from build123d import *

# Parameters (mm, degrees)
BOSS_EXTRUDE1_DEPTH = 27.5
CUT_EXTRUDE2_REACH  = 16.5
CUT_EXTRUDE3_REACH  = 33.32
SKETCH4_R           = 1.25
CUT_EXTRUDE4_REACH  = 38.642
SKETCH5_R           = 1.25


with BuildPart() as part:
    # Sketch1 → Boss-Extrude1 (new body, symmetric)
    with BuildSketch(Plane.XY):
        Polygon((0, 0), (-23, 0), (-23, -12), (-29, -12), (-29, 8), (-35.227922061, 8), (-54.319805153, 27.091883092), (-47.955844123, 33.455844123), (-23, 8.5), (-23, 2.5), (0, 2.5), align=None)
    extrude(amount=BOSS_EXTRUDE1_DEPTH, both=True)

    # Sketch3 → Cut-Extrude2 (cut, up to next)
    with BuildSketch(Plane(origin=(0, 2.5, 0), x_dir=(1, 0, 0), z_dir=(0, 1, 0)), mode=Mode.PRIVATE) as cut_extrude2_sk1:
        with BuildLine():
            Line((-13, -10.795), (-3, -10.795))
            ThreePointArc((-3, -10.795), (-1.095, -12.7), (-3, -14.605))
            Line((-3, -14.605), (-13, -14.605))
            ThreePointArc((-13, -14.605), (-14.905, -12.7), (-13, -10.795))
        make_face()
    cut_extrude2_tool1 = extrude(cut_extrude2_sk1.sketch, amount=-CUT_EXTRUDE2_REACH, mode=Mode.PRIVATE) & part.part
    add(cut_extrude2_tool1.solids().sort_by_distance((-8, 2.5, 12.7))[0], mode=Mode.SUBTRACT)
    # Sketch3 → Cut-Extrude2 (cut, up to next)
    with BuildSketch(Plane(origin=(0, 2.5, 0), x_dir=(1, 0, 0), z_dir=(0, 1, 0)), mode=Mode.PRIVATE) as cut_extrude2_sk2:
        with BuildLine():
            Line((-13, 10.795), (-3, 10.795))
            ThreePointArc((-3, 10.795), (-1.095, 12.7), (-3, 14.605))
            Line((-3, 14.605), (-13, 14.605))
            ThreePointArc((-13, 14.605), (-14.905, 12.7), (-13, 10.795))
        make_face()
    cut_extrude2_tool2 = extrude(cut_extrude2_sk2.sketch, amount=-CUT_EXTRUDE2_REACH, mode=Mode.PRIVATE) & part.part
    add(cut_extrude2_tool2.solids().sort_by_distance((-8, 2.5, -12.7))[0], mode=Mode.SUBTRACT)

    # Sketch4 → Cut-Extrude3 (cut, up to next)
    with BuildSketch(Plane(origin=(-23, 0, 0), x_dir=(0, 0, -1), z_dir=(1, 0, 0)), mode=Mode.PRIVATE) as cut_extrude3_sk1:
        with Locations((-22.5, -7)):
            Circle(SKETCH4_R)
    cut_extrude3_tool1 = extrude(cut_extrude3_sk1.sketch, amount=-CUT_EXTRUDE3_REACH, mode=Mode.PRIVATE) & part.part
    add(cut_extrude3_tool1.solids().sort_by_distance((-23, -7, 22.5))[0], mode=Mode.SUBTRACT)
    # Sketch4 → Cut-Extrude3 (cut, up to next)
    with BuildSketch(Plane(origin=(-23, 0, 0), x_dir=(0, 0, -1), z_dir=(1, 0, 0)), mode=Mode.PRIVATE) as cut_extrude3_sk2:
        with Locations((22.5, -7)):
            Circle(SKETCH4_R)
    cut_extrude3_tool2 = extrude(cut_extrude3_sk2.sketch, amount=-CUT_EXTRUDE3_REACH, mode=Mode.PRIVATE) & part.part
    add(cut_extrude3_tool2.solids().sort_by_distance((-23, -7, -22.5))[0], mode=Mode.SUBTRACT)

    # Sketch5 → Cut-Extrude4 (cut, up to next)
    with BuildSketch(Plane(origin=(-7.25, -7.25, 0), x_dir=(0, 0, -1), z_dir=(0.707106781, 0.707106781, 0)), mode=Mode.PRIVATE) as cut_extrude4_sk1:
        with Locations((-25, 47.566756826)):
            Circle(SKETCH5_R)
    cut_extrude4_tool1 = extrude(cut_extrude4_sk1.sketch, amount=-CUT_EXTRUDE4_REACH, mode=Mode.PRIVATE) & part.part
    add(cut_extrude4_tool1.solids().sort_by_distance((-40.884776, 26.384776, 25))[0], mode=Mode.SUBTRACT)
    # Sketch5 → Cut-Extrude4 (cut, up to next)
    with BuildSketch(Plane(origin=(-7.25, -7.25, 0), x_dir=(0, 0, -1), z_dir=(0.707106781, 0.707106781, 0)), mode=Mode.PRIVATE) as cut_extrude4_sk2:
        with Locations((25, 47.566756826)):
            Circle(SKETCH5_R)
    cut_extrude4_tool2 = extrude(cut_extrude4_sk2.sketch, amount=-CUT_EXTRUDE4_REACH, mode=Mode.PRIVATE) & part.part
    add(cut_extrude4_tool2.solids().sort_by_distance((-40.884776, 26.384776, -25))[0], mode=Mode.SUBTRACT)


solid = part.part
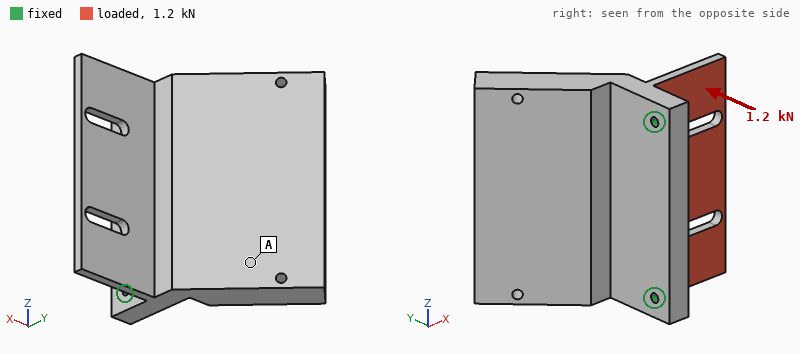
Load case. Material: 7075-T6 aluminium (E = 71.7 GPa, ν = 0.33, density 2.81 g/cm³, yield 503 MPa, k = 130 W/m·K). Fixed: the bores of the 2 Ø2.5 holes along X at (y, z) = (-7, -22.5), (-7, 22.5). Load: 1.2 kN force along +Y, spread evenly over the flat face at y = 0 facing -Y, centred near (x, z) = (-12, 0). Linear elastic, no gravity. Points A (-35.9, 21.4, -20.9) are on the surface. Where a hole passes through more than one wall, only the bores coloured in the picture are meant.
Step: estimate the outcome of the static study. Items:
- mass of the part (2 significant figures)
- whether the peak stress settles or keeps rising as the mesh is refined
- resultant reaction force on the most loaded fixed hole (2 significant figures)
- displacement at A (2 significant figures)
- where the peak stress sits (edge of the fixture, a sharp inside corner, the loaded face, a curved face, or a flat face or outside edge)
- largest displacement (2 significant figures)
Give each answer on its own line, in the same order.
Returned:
70 g
keeps rising
630 N
0.10 mm
edge of the fixture
0.48 mm
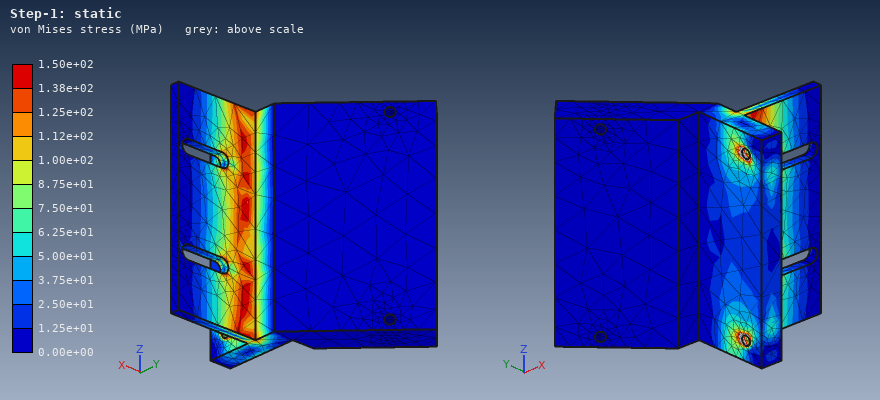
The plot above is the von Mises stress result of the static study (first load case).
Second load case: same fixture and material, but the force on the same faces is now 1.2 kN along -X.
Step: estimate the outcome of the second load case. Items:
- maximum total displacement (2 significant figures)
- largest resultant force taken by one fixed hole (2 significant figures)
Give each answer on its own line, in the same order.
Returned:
53 µm
610 N
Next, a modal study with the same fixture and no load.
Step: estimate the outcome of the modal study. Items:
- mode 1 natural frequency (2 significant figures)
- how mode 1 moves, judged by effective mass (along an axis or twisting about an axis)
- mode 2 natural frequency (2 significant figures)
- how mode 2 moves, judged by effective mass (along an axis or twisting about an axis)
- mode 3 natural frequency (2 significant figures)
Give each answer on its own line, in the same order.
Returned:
1400 Hz
along X
3800 Hz
along Y
4200 Hz
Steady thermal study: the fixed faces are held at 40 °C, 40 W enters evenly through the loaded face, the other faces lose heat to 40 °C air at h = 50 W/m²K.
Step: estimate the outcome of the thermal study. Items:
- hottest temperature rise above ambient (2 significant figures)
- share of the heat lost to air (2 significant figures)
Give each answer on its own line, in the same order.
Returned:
41 K
17 %
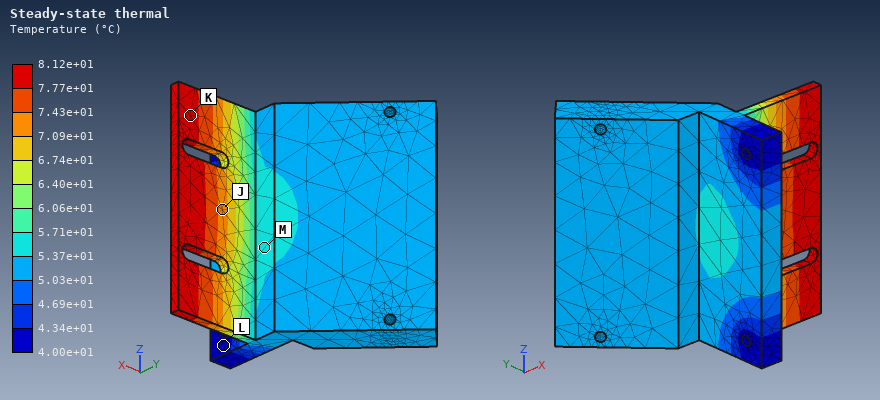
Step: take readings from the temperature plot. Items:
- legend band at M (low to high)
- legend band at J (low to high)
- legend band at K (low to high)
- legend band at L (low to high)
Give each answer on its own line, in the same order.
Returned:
5.37e+01 to 5.71e+01 °C
7.09e+01 to 7.43e+01 °C
7.77e+01 to 8.12e+01 °C
4.00e+01 to 4.34e+01 °C
